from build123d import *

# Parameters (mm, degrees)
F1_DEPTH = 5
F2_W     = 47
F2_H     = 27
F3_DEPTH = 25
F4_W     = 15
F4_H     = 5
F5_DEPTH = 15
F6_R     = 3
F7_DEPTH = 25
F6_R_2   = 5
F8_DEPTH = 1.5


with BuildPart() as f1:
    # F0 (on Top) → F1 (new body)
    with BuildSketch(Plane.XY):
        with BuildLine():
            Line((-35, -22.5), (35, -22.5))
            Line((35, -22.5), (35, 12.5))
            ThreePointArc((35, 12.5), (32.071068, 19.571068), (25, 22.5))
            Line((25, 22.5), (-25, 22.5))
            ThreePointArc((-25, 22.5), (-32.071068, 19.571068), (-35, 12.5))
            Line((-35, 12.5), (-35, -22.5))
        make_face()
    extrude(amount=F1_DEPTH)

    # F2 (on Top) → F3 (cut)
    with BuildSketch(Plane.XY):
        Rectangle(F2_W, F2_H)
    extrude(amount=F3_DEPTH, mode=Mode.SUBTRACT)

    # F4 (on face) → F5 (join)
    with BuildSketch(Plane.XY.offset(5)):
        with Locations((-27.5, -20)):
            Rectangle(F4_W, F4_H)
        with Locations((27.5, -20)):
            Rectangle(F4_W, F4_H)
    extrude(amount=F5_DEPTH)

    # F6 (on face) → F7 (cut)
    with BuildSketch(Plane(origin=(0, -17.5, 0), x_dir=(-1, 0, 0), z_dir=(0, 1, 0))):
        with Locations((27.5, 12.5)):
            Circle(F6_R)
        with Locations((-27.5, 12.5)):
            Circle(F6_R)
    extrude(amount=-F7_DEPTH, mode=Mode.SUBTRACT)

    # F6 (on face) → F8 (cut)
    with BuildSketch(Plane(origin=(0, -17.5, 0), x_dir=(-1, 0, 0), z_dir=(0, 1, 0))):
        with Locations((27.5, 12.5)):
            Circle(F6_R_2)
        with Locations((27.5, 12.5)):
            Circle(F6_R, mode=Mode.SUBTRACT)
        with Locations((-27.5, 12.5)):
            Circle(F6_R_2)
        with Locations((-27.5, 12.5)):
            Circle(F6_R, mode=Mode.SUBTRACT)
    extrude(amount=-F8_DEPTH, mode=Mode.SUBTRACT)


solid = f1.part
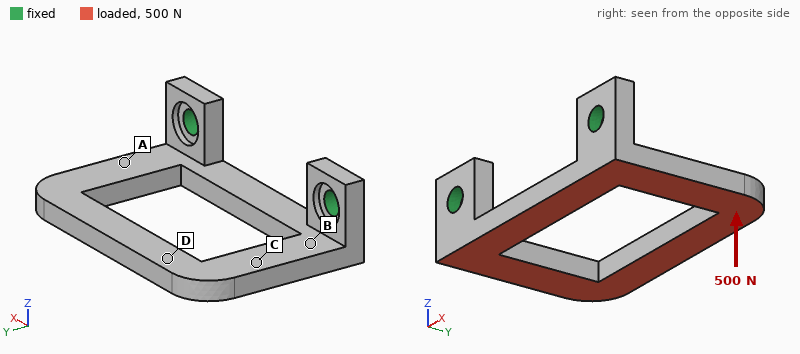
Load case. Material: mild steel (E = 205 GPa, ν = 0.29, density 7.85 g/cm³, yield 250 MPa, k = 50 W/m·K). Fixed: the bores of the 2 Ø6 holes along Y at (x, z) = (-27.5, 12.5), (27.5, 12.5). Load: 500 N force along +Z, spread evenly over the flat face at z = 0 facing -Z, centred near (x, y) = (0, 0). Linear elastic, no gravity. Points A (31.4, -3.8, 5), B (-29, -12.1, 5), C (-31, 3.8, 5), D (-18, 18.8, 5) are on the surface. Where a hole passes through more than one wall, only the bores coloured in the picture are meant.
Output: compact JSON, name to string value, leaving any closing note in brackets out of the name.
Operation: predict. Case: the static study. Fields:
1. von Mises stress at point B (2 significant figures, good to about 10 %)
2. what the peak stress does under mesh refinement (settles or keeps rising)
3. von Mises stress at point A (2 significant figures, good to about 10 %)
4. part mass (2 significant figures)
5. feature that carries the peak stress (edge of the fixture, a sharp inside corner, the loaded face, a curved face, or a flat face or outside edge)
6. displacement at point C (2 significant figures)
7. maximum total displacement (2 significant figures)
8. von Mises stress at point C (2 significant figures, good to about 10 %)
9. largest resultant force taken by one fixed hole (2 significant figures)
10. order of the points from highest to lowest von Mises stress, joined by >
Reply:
{"von Mises stress at point B": "68 MPa", "what the peak stress does under mesh refinement": "keeps rising", "von Mises stress at point A": "46 MPa", "part mass": "86 g", "feature that carries the peak stress": "edge of the fixture", "displacement at point C": "0.074 mm", "maximum total displacement": "0.17 mm", "von Mises stress at point C": "28 MPa", "largest resultant force taken by one fixed hole": "250 N", "order of the points from highest to lowest von Mises stress, joined by >": "B > A > C > D"}
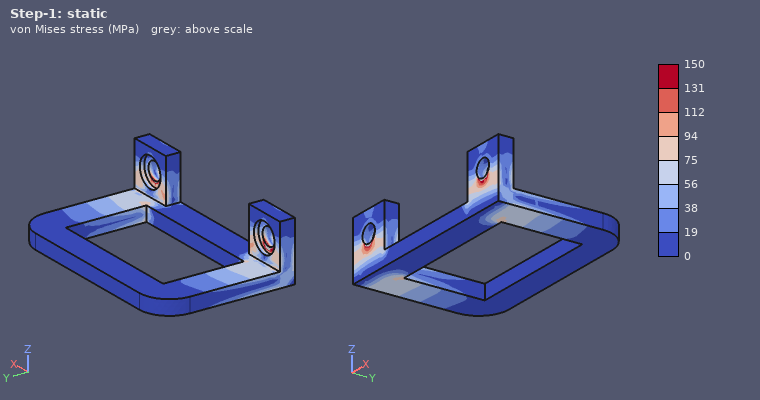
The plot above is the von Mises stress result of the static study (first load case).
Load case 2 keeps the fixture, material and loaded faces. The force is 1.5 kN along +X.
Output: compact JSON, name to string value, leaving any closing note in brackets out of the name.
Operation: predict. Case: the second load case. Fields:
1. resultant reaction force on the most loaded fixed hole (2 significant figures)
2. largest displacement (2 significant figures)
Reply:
{"resultant reaction force on the most loaded fixed hole": "850 N", "largest displacement": "51 µm"}
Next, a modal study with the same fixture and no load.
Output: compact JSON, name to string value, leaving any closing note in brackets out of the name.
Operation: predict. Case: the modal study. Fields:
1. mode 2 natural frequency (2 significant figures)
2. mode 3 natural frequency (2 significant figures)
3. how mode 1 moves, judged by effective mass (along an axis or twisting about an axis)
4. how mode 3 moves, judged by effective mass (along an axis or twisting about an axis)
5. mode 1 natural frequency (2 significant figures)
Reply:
{"mode 2 natural frequency": "2500 Hz", "mode 3 natural frequency": "3700 Hz", "how mode 1 moves, judged by effective mass": "along Z", "how mode 3 moves, judged by effective mass": "along X", "mode 1 natural frequency": "1200 Hz"}
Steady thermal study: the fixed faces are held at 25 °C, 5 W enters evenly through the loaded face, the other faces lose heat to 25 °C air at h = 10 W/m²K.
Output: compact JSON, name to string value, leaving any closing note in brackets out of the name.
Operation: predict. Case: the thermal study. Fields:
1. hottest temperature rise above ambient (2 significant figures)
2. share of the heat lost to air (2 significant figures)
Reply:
{"hottest temperature rise above ambient": "22 K", "share of the heat lost to air": "9.9 %"}
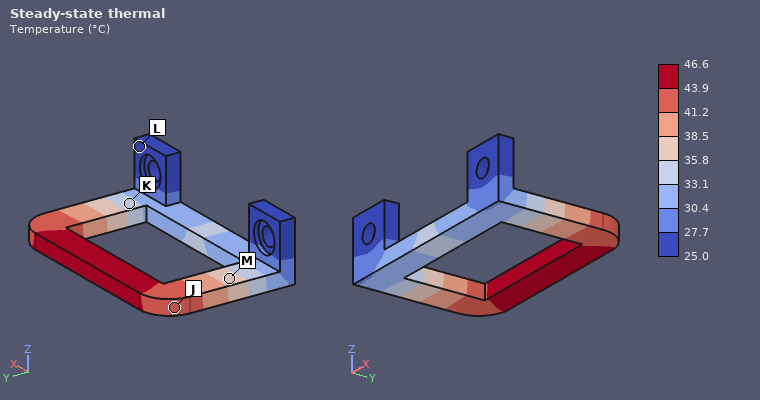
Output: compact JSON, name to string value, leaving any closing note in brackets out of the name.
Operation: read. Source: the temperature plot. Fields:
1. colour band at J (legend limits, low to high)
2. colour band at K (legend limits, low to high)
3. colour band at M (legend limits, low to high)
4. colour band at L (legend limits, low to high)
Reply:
{"colour band at J": "41.2 to 43.9 °C", "colour band at K": "33.1 to 35.8 °C", "colour band at M": "35.8 to 38.5 °C", "colour band at L": "25.0 to 27.7 °C"}
